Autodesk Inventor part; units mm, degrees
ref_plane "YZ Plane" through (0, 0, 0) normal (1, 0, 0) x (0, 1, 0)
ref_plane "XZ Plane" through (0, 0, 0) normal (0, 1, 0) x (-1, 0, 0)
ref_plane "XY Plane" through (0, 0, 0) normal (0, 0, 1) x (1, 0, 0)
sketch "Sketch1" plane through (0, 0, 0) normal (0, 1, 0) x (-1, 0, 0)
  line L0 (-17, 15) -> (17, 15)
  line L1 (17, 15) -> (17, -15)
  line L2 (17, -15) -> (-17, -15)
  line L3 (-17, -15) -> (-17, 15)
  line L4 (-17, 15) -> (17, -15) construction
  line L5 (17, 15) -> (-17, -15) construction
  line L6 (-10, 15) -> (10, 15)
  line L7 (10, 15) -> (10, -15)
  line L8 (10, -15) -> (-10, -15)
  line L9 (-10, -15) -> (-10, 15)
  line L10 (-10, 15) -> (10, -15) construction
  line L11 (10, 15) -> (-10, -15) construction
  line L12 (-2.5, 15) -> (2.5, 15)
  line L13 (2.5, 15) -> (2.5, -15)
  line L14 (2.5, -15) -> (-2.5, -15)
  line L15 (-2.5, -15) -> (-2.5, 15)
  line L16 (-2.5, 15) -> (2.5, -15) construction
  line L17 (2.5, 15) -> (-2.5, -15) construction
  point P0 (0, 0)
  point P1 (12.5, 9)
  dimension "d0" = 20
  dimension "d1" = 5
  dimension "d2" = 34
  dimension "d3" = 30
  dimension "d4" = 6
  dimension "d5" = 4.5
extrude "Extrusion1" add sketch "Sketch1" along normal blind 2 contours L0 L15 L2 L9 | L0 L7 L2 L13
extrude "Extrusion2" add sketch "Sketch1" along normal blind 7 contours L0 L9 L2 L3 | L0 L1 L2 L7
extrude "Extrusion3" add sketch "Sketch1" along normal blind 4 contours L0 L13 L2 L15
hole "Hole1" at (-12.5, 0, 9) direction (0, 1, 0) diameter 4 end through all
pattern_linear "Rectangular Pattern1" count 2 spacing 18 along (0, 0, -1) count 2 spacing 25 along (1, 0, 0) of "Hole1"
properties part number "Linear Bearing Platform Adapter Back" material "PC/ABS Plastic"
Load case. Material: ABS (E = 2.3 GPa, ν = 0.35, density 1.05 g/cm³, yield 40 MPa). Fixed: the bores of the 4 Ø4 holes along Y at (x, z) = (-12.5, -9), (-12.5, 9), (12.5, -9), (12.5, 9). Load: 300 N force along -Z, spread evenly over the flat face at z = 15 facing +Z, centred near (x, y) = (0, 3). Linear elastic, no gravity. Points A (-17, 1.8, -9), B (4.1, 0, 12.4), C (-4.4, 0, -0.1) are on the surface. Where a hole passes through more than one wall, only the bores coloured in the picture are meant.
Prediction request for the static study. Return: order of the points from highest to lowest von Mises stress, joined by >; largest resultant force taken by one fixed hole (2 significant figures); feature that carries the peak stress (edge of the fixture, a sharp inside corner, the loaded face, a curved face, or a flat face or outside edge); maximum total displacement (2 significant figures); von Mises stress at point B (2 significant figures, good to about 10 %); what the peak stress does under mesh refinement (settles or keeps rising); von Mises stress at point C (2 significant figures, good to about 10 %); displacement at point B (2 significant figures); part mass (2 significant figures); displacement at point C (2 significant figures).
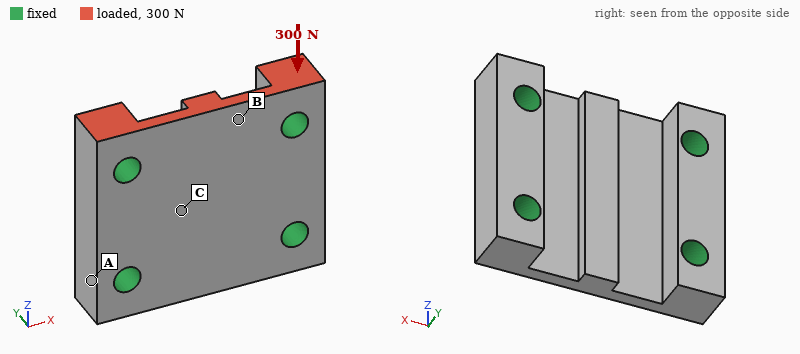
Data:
B > C > A
130 N
edge of the fixture
22 µm
1.7 MPa
keeps rising
1.1 MPa
13 µm
4.3 g
5.8 µm
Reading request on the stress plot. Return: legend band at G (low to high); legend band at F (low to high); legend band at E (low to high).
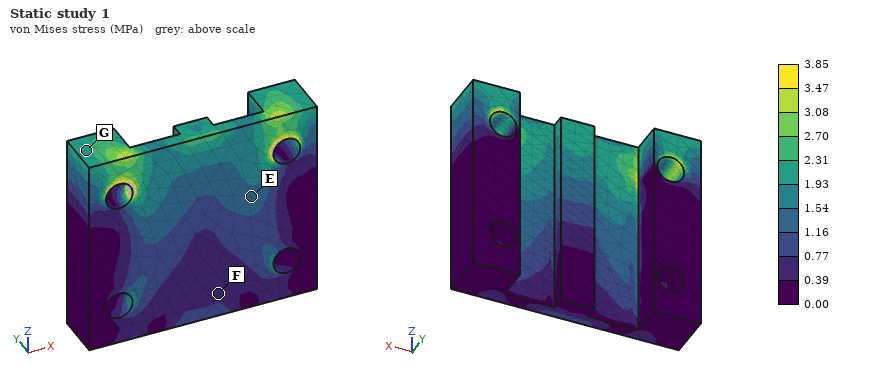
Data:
1.93 to 2.31 MPa
0.39 to 0.77 MPa
1.16 to 1.54 MPa
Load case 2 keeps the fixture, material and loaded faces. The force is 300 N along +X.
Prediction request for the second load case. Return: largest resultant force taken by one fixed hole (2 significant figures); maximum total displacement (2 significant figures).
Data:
150 N
31 µm
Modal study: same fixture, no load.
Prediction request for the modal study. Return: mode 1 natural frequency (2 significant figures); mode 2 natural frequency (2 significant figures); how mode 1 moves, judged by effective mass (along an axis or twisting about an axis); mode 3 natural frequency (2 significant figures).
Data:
5800 Hz
6200 Hz
along Y
9500 Hz
